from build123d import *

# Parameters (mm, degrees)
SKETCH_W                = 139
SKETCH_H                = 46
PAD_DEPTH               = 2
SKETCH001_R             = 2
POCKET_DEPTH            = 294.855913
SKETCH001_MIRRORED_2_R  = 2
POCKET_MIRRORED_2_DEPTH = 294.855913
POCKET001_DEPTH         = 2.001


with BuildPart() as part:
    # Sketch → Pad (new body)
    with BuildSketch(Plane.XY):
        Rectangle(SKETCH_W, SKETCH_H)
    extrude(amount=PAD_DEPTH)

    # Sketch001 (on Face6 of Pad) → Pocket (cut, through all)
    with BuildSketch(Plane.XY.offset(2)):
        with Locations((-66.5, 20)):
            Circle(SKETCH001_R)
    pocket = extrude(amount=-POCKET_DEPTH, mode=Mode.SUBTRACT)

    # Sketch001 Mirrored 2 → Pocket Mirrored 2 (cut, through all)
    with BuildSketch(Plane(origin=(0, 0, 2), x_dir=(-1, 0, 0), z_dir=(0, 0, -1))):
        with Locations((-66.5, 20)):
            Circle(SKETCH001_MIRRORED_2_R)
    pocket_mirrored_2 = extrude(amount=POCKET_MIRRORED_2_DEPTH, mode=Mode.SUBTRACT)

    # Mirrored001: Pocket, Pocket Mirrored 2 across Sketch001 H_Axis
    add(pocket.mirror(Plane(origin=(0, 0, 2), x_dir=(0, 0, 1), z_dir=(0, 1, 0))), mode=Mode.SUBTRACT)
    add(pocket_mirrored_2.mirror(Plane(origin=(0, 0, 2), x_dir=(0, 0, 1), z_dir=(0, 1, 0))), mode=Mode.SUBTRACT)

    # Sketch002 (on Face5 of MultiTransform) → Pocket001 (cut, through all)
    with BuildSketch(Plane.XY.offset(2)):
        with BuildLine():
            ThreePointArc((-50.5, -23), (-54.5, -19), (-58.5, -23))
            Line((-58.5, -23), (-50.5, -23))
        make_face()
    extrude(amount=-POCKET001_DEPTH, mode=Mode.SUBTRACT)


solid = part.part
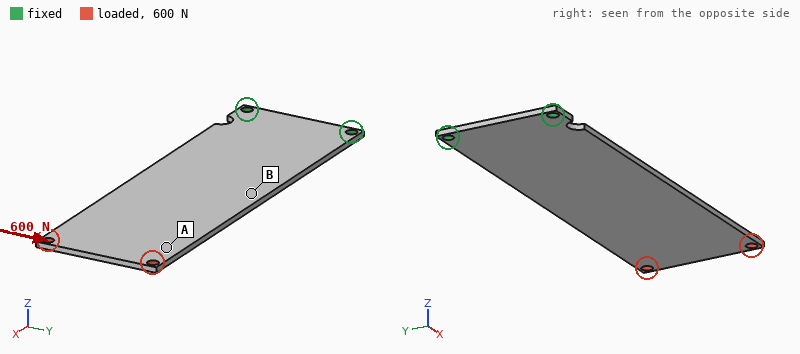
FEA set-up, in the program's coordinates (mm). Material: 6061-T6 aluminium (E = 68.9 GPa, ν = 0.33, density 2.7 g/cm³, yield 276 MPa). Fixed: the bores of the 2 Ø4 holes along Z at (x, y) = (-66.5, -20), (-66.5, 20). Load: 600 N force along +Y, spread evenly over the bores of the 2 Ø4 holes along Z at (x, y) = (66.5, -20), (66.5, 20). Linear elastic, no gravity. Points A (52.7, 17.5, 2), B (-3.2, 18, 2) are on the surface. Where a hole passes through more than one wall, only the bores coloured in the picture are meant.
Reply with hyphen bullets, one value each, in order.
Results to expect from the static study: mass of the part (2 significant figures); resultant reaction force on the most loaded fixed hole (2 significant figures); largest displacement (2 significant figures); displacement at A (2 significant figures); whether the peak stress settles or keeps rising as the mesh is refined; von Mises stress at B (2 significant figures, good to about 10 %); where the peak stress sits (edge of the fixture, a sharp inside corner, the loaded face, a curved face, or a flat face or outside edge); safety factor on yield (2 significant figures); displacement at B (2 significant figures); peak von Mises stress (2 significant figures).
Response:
- 34 g
- 2.1 kN
- 0.55 mm
- 0.45 mm
- settles
- 47 MPa
- a curved face
- 0.83
- 0.18 mm
- 330 MPa
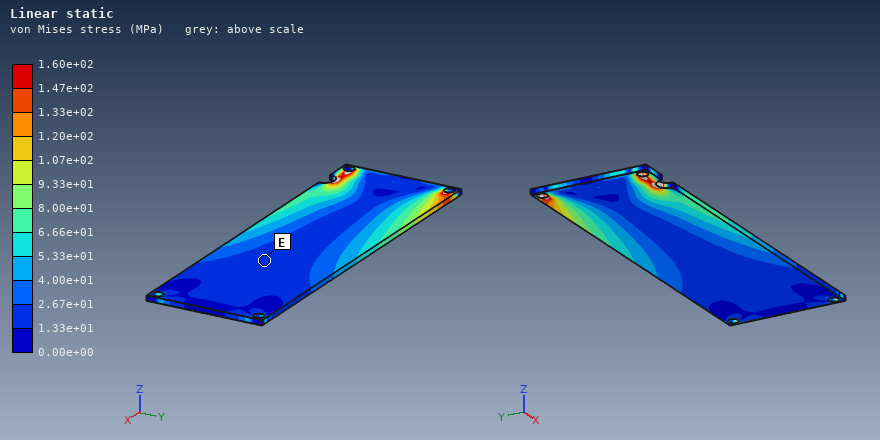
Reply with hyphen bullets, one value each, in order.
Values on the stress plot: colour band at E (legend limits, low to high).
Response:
- 1.33e+01 to 2.67e+01 MPa
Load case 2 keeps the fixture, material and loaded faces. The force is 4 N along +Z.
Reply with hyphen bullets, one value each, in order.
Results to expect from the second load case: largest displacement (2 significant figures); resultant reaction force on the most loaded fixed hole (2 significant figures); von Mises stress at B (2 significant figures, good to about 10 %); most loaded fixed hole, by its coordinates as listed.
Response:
- 1.7 mm
- 2.2 N
- 9.2 MPa
- (-66.5, 20)
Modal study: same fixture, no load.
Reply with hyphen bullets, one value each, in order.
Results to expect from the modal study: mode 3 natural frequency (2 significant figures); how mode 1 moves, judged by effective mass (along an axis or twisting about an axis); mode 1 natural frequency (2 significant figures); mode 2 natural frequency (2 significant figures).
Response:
- 540 Hz
- along Z
- 83 Hz
- 530 Hz
